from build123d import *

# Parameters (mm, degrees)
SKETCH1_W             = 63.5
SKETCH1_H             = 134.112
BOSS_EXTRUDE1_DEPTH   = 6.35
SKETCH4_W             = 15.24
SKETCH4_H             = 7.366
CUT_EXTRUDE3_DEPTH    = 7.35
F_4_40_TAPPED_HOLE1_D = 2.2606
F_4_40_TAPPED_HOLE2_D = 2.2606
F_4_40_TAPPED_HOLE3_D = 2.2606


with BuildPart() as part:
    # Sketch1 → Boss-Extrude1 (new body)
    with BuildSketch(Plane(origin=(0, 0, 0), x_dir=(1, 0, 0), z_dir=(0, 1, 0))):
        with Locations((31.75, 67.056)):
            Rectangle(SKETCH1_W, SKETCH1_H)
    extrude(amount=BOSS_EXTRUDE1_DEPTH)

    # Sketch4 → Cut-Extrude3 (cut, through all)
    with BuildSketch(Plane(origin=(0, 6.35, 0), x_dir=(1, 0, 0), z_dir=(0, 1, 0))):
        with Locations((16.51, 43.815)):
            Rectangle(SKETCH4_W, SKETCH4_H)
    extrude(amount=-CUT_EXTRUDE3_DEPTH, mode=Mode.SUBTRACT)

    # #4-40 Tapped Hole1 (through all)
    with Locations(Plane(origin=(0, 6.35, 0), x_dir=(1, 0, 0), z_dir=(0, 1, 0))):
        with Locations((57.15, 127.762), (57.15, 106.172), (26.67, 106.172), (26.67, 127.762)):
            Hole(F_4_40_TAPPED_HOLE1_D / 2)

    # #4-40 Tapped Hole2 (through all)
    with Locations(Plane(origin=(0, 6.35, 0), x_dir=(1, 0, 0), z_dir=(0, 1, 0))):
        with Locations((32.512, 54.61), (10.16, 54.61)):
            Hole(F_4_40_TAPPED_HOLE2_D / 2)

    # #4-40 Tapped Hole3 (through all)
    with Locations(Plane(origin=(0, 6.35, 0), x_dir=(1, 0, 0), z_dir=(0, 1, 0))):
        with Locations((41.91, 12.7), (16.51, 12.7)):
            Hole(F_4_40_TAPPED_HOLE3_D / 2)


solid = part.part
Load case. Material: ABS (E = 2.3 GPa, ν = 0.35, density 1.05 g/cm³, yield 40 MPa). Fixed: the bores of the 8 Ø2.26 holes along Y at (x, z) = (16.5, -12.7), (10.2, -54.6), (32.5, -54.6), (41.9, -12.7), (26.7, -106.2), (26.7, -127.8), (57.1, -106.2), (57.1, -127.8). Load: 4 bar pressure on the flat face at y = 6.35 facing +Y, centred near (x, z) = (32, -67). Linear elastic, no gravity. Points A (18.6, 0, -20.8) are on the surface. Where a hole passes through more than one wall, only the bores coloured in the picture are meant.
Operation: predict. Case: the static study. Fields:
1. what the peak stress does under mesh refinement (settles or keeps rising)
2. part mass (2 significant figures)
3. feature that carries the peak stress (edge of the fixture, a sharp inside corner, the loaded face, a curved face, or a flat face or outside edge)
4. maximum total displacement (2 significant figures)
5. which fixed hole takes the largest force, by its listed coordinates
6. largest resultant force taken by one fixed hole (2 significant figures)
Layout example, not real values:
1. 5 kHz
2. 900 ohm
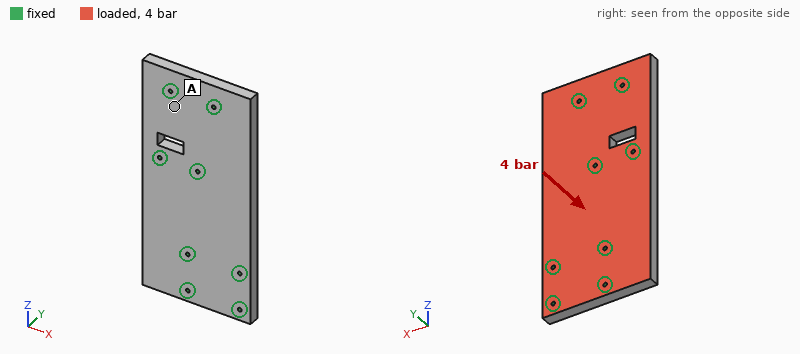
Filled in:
1. keeps rising
2. 56 g
3. edge of the fixture
4. 0.95 mm
5. (32.5, -54.6)
6. 800 N
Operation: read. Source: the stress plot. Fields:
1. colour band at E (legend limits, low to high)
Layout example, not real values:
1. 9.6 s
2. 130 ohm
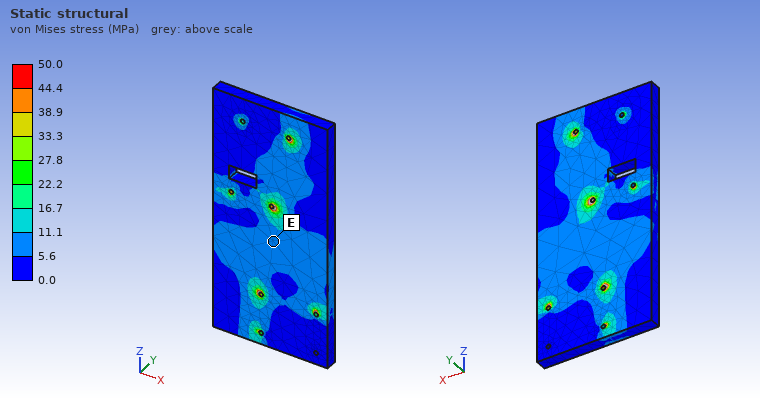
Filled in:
1. 5.6 to 11.1 MPa
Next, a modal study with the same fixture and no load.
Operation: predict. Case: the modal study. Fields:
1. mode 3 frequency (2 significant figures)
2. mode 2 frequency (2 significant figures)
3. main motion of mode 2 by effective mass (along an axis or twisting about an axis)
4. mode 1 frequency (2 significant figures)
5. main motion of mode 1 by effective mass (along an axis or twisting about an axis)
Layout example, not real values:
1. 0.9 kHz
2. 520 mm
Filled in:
1. 2500 Hz
2. 1900 Hz
3. along Y
4. 1600 Hz
5. along Y
